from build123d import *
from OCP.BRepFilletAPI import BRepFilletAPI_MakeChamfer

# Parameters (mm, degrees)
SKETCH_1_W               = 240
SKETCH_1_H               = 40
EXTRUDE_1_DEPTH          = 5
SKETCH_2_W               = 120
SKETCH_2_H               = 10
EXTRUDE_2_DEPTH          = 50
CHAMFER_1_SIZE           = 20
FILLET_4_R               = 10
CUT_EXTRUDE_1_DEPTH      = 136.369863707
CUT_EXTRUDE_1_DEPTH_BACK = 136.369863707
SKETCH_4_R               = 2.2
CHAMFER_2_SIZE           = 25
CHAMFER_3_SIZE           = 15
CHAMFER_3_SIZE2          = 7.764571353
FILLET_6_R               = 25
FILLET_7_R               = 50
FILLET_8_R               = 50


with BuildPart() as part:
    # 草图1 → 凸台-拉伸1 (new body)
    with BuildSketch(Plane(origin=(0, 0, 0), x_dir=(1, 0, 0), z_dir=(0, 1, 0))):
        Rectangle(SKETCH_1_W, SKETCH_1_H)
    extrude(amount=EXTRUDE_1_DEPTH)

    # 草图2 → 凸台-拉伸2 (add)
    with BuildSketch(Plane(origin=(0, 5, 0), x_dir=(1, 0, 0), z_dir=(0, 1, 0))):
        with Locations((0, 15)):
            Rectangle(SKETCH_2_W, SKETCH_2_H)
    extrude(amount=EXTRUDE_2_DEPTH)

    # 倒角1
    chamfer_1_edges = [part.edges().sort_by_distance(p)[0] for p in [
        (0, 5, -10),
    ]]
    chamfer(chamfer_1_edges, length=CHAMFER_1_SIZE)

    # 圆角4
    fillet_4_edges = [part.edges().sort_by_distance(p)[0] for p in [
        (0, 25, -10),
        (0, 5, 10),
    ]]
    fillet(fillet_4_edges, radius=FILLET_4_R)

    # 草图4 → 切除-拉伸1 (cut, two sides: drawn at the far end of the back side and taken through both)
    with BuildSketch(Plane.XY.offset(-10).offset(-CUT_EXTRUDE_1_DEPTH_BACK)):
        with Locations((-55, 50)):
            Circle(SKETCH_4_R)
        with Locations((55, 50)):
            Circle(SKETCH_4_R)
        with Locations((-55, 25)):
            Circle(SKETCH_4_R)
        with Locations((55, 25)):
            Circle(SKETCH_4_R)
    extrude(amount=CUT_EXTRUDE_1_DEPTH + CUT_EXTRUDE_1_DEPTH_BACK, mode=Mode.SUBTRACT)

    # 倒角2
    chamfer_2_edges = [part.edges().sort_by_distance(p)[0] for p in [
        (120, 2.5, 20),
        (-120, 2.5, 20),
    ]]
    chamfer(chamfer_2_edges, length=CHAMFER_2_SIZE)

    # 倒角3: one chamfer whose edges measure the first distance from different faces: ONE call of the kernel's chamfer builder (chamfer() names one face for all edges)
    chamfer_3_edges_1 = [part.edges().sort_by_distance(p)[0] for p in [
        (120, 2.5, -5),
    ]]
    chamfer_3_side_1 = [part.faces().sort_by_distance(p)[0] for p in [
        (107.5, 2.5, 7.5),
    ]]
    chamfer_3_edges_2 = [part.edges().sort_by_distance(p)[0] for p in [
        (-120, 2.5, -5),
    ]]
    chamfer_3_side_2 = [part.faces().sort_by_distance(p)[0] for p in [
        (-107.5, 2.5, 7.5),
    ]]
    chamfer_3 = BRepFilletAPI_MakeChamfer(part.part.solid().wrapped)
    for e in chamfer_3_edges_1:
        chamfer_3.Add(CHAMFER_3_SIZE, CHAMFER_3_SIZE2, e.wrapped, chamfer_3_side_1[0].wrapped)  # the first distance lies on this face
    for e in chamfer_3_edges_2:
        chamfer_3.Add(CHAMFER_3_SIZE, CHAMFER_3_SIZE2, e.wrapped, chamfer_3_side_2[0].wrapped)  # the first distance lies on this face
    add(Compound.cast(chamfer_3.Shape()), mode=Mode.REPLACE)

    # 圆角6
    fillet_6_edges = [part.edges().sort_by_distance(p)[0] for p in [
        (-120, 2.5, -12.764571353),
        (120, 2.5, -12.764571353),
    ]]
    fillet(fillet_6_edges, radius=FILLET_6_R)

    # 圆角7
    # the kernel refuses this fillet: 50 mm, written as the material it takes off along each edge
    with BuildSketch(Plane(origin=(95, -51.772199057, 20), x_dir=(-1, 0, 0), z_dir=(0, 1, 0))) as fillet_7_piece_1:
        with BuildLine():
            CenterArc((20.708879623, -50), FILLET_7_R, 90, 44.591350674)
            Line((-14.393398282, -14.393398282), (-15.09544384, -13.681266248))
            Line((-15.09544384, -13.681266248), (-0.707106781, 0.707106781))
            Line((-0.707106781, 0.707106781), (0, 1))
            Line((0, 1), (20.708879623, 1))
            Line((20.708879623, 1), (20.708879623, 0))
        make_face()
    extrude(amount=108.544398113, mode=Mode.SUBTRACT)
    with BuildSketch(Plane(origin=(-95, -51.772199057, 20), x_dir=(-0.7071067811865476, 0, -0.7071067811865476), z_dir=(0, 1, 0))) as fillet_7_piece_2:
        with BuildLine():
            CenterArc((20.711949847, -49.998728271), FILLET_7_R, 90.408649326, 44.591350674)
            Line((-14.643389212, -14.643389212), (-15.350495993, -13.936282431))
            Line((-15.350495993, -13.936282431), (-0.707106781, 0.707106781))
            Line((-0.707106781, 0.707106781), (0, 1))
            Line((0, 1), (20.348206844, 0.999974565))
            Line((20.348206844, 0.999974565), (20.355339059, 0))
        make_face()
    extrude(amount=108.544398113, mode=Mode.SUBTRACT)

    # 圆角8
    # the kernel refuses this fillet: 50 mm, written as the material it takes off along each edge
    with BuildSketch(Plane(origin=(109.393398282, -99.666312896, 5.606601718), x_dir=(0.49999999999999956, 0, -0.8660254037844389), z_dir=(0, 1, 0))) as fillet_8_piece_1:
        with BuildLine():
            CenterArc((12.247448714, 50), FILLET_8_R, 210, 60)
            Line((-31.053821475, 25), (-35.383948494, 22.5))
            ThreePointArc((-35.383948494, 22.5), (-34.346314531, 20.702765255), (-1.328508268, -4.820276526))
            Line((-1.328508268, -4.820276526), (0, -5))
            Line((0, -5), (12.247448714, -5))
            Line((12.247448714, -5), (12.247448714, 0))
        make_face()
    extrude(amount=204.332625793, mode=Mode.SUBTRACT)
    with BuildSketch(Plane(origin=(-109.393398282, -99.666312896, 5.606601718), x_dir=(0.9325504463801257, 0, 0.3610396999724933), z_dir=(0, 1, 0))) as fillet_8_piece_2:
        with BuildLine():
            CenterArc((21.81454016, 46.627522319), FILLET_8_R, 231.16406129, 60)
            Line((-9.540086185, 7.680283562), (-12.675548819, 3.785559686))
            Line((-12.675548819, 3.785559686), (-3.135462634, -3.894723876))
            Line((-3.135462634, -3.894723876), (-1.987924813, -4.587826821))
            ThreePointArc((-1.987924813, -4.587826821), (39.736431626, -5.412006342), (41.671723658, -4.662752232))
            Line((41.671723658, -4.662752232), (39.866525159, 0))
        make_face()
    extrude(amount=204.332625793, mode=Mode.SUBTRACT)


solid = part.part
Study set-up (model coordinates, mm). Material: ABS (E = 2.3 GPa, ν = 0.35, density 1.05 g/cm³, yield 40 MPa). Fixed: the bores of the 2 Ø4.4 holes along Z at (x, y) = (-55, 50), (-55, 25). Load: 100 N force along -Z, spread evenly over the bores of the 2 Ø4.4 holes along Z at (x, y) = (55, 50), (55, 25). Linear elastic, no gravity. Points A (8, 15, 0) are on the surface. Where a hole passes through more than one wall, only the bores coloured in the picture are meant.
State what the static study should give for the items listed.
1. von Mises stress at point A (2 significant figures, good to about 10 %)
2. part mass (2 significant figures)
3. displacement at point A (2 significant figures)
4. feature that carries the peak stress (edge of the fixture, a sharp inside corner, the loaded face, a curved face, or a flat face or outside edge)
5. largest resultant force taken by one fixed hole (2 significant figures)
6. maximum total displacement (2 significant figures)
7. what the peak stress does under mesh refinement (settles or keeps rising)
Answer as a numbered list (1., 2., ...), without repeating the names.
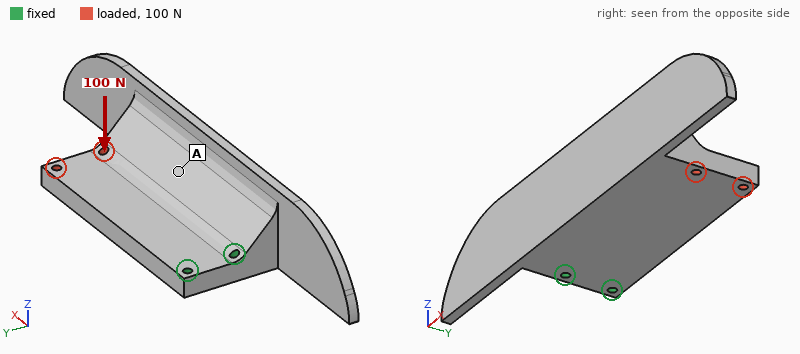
1. 1.6 MPa
2. 130 g
3. 0.97 mm
4. edge of the fixture
5. 69 N
6. 2.9 mm
7. keeps rising
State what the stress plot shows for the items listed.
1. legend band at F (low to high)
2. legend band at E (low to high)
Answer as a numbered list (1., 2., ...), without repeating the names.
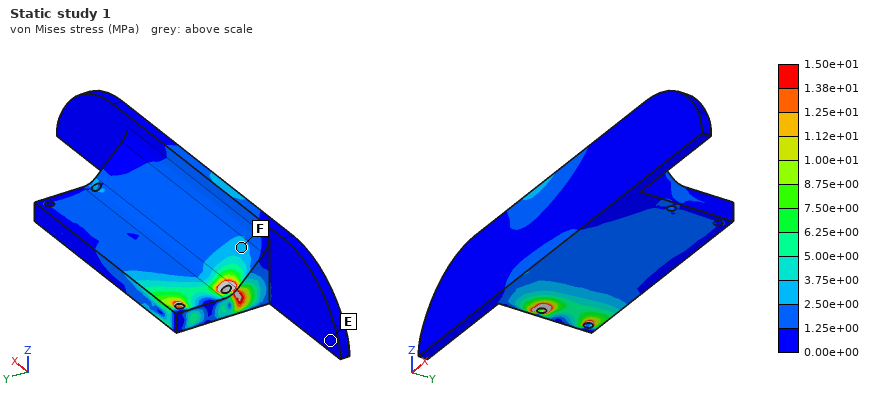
1. 2.50e+00 to 3.75e+00 MPa
2. 0.00e+00 to 1.25e+00 MPa
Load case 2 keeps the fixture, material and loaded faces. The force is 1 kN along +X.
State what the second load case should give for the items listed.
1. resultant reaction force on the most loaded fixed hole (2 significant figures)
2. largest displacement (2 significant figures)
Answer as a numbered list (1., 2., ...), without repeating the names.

1. 520 N
2. 0.35 mm
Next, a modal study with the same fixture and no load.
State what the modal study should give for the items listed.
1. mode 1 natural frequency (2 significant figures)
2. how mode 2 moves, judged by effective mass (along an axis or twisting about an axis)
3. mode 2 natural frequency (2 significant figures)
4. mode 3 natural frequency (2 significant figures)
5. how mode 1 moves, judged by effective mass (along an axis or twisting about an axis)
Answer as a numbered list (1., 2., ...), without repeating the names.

1. 150 Hz
2. along Y
3. 320 Hz
4. 390 Hz
5. along Z
